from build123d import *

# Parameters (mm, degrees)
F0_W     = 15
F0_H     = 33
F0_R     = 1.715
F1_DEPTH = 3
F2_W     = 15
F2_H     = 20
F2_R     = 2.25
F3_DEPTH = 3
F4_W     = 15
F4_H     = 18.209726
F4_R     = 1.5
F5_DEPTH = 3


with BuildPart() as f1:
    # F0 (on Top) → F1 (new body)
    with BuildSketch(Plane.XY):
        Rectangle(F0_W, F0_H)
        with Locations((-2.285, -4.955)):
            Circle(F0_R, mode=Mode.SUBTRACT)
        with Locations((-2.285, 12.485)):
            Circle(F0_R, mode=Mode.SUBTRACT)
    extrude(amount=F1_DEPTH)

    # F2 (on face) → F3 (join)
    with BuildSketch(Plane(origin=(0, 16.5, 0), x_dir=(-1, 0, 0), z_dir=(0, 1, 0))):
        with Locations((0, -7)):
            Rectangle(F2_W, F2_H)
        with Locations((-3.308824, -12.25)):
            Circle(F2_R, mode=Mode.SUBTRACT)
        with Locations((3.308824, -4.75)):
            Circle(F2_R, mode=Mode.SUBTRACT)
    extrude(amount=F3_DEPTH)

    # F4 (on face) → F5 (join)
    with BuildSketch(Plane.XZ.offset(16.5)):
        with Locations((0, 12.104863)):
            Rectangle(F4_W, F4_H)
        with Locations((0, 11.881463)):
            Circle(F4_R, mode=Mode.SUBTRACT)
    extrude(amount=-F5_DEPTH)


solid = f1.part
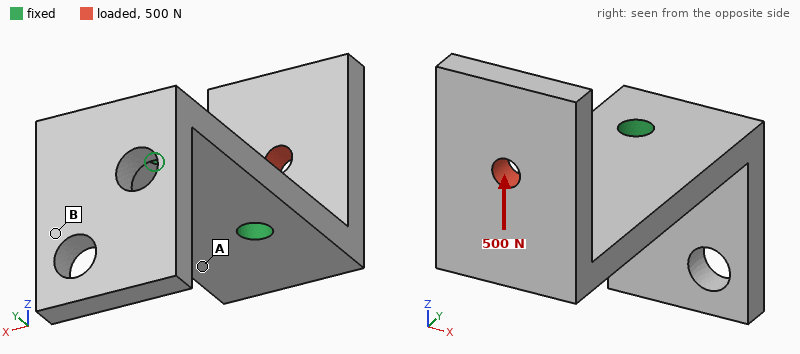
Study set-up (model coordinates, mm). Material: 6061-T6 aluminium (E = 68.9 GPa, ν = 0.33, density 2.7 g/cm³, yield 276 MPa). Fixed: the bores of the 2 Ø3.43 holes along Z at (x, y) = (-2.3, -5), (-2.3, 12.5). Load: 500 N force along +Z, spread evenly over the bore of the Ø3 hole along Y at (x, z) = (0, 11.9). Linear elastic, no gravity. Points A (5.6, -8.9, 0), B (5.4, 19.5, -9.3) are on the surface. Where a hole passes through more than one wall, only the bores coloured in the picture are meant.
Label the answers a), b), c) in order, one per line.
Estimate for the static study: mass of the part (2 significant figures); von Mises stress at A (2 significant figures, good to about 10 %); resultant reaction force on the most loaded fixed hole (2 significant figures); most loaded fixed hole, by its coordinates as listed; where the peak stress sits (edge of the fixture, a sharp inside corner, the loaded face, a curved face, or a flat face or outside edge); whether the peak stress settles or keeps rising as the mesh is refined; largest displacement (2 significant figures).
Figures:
a) 8.2 g
b) 92 MPa
c) 560 N
d) (-2.3, -5)
e) edge of the fixture
f) keeps rising
g) 0.23 mm
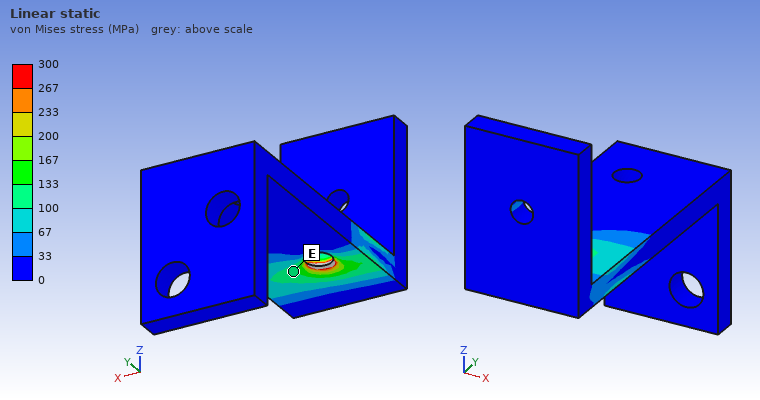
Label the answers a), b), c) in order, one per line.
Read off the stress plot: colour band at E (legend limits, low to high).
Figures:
a) 100 to 133 MPa
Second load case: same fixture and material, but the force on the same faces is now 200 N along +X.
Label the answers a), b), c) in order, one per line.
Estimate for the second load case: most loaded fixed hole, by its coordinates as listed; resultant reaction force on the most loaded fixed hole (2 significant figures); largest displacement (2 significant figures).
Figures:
a) (-2.3, -5)
b) 280 N
c) 0.12 mm
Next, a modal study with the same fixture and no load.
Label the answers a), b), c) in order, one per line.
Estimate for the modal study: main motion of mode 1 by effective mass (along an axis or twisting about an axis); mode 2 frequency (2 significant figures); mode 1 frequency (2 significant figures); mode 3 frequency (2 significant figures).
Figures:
a) along Y
b) 5100 Hz
c) 3600 Hz
d) 5200 Hz
